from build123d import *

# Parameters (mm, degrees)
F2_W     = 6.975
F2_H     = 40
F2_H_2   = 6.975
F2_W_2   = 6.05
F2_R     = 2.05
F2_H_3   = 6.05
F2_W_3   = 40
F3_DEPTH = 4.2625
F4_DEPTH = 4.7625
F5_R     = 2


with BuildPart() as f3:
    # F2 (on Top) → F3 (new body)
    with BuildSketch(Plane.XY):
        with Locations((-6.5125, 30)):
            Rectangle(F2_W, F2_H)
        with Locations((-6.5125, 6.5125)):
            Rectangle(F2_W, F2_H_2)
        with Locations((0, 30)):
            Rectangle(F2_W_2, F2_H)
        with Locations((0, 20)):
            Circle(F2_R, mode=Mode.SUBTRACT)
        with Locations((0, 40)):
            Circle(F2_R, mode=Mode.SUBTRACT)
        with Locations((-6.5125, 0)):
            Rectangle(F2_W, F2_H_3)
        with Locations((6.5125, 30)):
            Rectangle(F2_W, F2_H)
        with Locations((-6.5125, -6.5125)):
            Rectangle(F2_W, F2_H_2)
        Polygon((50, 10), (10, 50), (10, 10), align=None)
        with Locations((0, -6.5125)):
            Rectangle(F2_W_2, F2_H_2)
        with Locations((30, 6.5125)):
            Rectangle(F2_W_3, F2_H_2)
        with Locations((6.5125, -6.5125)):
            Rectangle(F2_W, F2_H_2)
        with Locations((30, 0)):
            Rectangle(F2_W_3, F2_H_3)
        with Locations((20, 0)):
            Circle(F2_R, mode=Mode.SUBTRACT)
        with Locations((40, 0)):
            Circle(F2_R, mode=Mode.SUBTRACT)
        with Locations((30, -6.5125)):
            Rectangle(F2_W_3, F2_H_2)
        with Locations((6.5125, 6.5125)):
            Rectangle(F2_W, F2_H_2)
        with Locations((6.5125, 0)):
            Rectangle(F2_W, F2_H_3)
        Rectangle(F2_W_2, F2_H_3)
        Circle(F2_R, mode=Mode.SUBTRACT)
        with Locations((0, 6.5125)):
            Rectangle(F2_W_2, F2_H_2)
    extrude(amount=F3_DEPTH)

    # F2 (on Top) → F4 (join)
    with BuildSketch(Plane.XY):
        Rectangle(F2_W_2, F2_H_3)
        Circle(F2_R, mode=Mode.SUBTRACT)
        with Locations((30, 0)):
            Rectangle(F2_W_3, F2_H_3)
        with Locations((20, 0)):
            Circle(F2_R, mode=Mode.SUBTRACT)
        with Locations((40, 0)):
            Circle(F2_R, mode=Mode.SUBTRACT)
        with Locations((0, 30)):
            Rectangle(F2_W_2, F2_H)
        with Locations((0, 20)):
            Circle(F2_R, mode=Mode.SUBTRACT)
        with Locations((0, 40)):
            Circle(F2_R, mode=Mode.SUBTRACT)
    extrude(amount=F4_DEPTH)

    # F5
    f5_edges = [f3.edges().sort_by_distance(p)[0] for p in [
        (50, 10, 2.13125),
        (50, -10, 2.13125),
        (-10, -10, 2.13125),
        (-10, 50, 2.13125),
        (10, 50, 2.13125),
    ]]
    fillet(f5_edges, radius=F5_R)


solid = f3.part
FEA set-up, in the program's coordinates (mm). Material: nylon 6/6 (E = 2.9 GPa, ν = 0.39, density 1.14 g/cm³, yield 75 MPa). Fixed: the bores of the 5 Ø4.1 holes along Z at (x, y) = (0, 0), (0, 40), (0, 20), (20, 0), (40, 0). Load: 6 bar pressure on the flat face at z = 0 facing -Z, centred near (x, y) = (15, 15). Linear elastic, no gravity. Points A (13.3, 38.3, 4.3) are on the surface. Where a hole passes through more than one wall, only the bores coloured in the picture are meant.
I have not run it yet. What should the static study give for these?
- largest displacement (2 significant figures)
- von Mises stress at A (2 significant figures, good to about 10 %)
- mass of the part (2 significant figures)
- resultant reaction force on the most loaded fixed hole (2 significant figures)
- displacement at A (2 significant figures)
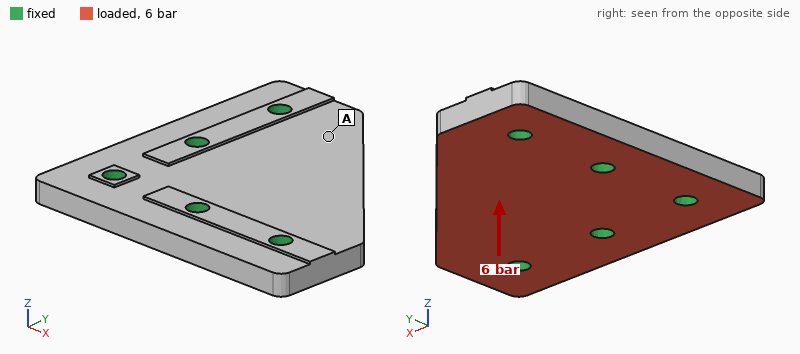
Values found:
0.91 mm
7.5 MPa
14 g
380 N
0.36 mm
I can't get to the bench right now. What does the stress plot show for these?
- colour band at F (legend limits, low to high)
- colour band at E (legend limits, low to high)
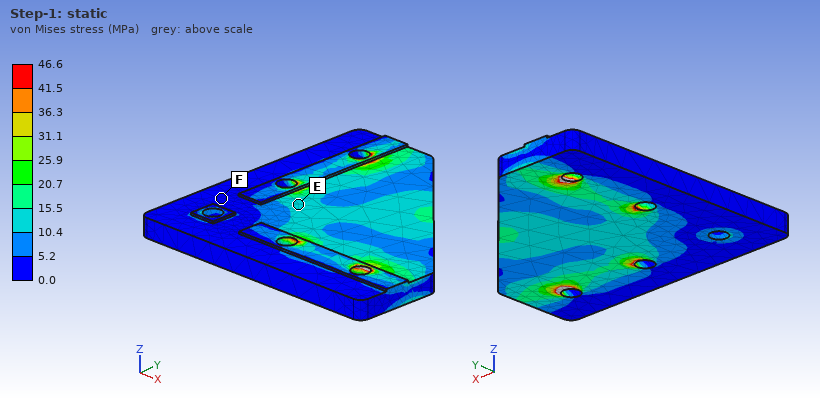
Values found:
0.0 to 5.2 MPa
10.4 to 15.5 MPa
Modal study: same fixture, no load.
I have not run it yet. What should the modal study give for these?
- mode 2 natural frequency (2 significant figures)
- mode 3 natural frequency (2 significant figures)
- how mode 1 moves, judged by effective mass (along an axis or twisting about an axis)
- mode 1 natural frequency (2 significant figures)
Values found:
5100 Hz
7000 Hz
along Z
2500 Hz
